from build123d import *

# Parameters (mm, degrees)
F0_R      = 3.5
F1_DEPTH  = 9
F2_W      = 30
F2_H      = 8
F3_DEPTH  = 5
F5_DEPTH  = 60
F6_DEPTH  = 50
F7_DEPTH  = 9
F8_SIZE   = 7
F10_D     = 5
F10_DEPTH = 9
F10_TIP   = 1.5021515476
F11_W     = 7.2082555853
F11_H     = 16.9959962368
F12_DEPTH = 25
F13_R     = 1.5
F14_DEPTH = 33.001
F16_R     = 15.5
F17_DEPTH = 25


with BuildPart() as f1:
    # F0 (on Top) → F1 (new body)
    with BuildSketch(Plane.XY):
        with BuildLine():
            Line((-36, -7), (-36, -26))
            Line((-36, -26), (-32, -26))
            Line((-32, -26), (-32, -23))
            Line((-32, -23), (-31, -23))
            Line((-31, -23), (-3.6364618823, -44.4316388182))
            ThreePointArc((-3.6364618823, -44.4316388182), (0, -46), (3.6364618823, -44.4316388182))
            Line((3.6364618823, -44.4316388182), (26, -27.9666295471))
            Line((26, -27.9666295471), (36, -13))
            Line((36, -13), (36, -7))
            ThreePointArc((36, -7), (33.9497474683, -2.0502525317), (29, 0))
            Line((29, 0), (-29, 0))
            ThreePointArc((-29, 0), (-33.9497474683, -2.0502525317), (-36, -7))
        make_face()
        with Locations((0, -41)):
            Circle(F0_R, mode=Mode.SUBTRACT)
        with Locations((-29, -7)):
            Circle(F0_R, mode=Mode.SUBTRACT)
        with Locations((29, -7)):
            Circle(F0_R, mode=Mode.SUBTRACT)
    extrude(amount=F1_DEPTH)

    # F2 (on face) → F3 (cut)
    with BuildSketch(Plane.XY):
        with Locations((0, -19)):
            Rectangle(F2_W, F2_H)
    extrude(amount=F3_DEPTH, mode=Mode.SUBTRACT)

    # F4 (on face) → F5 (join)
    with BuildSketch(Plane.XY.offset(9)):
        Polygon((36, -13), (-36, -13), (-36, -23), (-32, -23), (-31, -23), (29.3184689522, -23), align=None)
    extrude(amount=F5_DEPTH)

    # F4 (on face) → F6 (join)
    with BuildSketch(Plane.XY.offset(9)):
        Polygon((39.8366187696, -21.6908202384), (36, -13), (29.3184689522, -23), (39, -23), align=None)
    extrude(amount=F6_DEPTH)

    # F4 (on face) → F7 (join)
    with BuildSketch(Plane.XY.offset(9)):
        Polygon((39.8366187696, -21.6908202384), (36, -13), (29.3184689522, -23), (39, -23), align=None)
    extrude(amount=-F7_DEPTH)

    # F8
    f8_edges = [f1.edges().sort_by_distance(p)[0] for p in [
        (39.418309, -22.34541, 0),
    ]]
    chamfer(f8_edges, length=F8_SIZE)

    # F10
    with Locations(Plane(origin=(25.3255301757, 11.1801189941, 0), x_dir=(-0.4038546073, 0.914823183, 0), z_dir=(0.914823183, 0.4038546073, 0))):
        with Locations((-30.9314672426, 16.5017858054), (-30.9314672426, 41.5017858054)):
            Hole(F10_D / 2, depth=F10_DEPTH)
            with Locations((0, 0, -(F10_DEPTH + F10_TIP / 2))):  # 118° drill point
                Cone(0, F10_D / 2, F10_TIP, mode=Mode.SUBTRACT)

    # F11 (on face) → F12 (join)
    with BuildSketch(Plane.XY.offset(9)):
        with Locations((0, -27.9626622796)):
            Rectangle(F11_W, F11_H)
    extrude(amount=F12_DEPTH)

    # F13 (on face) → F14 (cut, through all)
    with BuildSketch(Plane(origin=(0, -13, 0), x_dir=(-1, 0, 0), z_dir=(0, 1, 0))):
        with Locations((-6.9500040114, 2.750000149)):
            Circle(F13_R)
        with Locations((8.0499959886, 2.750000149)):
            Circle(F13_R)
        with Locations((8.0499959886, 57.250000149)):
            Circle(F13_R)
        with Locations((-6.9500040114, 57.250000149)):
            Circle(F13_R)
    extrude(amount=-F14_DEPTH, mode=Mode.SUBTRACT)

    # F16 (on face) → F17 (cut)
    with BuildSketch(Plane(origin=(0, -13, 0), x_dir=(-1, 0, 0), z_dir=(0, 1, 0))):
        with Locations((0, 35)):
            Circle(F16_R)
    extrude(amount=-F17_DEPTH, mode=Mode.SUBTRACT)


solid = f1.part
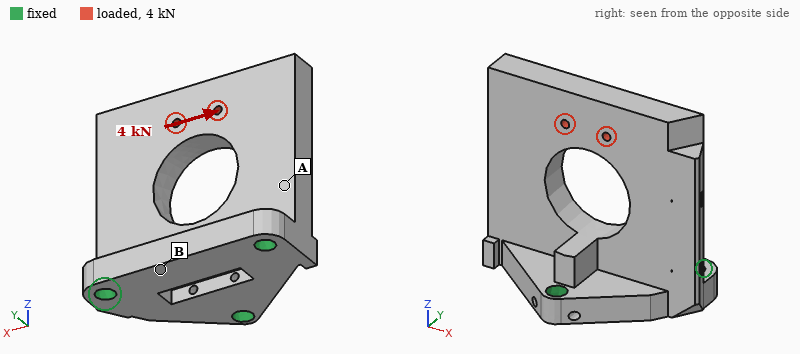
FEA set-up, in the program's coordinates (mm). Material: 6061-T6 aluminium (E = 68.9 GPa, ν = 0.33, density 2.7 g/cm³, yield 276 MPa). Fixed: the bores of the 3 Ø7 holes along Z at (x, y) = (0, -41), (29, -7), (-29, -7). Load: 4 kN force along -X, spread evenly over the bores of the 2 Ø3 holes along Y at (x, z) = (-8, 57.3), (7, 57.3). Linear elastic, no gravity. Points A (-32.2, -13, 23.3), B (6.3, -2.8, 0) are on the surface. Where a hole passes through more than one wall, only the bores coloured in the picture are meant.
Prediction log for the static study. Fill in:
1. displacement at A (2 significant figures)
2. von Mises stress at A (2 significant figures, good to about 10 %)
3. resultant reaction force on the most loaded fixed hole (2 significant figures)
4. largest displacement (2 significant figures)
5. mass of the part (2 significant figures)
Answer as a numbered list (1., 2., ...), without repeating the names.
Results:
1. 32 µm
2. 33 MPa
3. 3.8 kN
4. 92 µm
5. 150 g
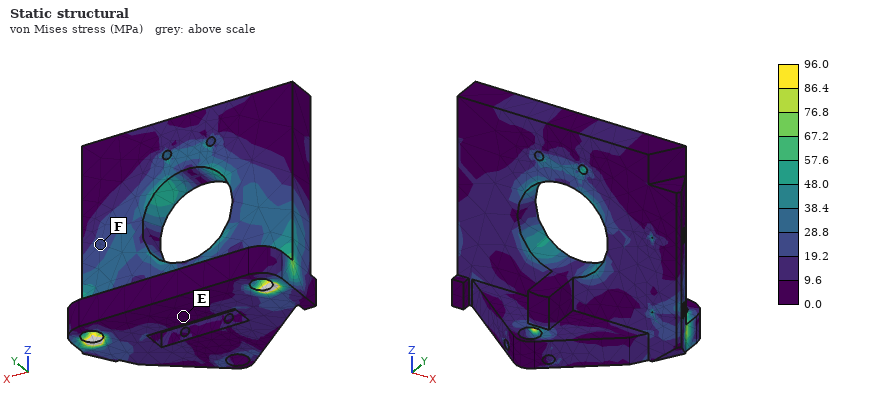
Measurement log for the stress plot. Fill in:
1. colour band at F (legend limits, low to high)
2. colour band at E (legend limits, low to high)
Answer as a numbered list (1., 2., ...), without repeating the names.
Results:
1. 19.2 to 28.8 MPa
2. 0.0 to 9.6 MPa
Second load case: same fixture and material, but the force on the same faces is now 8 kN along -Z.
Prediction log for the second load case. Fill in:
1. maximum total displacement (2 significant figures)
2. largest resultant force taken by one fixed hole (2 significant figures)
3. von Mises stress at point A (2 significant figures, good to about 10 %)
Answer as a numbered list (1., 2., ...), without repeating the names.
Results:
1. 62 µm
2. 3.4 kN
3. 18 MPa
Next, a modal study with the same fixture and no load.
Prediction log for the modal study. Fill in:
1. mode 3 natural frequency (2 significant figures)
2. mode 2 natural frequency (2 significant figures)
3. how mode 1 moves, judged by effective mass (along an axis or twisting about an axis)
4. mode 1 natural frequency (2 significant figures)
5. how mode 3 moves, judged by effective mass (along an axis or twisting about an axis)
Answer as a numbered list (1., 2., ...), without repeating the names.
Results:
1. 5300 Hz
2. 3400 Hz
3. along Y
4. 1700 Hz
5. along X
